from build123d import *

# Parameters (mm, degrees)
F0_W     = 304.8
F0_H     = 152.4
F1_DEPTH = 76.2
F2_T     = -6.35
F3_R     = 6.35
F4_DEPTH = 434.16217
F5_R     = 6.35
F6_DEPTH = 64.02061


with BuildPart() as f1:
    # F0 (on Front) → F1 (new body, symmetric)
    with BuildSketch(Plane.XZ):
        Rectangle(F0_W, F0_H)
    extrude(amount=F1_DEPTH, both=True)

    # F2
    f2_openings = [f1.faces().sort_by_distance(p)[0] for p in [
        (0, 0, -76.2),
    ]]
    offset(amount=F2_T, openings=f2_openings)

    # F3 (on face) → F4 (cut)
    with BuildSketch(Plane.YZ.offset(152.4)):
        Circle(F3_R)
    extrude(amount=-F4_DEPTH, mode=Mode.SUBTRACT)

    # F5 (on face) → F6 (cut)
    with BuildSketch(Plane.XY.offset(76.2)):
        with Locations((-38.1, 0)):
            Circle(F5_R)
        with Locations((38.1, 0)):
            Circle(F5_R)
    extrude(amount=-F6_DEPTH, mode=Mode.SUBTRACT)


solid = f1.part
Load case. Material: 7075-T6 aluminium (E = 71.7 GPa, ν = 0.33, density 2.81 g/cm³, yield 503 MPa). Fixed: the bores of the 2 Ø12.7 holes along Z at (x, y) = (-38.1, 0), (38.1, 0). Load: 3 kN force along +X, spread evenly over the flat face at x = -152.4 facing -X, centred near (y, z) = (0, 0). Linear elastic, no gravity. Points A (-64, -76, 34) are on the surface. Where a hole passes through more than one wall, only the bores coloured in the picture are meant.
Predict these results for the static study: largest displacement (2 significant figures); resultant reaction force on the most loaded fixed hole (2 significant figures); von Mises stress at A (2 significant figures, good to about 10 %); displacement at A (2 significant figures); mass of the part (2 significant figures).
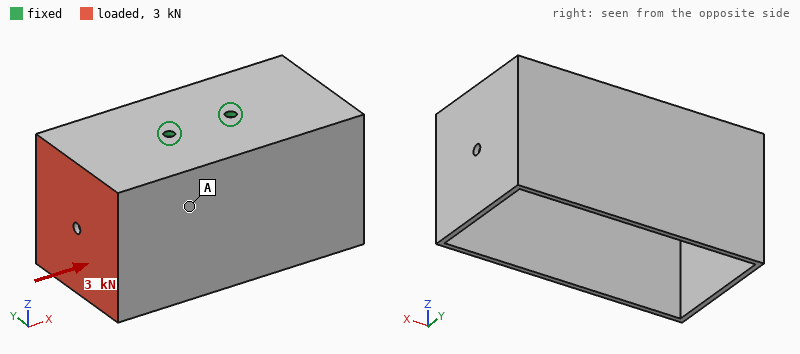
1.1 mm
2.6 kN
7.4 MPa
0.31 mm
3.1 kg
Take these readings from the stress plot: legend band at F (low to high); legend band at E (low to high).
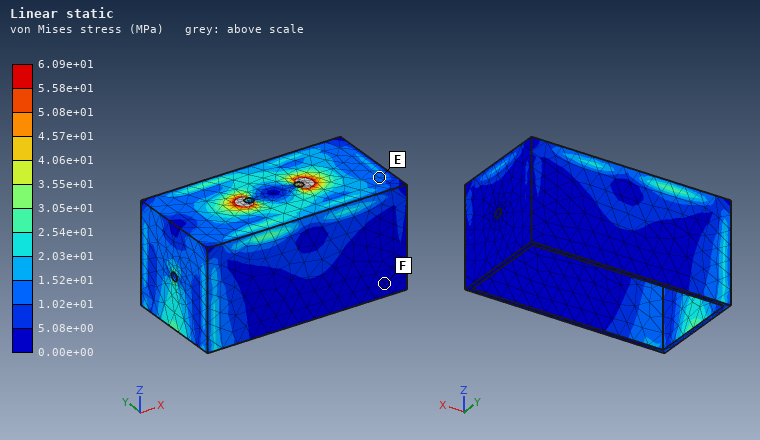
0.00e+00 to 5.08e+00 MPa
1.02e+01 to 1.52e+01 MPa
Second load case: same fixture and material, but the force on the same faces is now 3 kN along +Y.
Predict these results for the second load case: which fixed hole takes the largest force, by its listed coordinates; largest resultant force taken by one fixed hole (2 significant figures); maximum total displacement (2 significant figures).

(-38.1, 0)
6.9 kN
2.7 mm
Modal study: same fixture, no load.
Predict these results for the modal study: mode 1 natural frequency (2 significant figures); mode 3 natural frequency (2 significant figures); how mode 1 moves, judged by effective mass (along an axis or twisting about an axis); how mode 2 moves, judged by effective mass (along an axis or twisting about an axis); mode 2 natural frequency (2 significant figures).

130 Hz
230 Hz
along Y
along X
160 Hz
